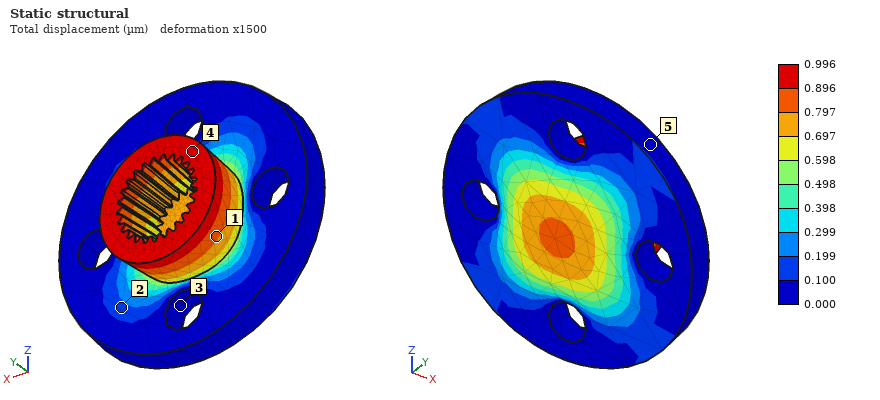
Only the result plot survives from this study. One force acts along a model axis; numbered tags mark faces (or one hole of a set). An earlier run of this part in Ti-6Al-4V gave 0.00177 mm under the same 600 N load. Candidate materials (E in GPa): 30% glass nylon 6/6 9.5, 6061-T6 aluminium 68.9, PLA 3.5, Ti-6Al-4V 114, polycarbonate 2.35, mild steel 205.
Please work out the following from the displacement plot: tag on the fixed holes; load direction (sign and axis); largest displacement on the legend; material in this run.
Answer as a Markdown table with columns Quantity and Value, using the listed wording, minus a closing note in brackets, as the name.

| Quantity | Value |
|---|---|
| tag on the fixed holes | 3 |
| load direction | -Y |
| largest displacement on the legend | 0.996 µm |
| material in this run | mild steel |
